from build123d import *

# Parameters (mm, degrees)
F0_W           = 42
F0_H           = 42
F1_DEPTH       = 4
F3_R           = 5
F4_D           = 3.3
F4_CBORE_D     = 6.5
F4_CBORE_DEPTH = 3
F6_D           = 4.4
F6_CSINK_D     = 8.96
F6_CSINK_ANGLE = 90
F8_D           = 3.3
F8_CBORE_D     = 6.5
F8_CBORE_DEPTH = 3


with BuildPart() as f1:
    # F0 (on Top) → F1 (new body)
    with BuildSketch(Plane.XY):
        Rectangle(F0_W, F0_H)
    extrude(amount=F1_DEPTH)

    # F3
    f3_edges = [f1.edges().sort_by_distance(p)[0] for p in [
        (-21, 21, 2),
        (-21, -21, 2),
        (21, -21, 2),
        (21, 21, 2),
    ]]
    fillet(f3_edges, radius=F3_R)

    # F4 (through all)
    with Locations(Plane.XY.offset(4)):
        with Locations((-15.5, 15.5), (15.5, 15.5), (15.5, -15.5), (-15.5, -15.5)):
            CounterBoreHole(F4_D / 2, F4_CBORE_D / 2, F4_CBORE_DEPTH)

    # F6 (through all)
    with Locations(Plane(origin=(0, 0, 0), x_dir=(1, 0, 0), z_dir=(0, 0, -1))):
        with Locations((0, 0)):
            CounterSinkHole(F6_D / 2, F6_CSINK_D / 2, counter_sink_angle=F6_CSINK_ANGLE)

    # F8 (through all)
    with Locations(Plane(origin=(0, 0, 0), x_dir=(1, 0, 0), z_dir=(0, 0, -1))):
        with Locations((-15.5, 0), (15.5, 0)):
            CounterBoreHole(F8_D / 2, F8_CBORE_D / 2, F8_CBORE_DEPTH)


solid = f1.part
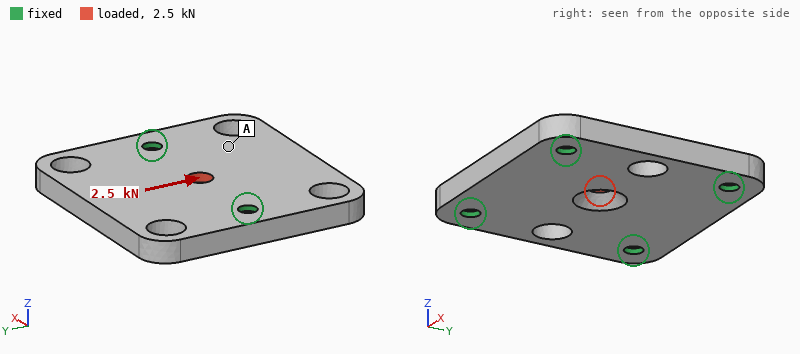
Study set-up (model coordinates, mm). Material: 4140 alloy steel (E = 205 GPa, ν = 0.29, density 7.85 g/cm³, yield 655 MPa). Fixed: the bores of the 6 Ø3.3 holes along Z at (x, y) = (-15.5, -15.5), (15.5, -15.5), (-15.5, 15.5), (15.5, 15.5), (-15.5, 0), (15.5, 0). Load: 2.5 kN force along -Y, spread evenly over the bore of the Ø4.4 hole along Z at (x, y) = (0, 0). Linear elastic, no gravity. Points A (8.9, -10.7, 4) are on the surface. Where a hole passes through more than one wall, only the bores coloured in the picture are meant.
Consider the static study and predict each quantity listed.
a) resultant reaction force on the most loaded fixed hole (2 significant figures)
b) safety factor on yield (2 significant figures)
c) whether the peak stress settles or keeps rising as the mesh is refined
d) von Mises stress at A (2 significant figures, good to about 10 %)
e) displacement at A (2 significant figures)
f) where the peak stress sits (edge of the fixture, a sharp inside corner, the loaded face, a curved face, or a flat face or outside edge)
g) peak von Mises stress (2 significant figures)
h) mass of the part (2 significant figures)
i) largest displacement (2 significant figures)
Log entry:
510 N
3.3
settles
14 MPa
1.5 µm
the loaded face
200 MPa
49 g
4.2 µm
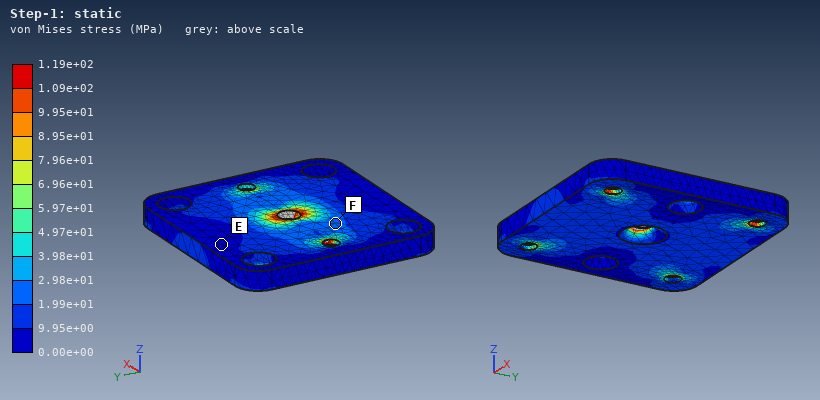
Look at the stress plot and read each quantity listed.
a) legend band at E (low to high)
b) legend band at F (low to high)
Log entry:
0.00e+00 to 9.95e+00 MPa
1.99e+01 to 2.98e+01 MPa
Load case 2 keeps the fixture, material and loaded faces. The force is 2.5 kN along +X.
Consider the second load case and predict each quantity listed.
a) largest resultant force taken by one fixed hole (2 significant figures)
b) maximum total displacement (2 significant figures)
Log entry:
580 N
3.6 µm
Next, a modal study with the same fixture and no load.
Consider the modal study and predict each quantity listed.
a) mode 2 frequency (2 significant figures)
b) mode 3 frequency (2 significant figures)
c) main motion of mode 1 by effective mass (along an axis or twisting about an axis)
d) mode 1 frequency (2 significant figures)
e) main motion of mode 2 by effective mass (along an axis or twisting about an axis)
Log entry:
15 kHz
22 kHz
along Z
13 kHz
twisting about X
